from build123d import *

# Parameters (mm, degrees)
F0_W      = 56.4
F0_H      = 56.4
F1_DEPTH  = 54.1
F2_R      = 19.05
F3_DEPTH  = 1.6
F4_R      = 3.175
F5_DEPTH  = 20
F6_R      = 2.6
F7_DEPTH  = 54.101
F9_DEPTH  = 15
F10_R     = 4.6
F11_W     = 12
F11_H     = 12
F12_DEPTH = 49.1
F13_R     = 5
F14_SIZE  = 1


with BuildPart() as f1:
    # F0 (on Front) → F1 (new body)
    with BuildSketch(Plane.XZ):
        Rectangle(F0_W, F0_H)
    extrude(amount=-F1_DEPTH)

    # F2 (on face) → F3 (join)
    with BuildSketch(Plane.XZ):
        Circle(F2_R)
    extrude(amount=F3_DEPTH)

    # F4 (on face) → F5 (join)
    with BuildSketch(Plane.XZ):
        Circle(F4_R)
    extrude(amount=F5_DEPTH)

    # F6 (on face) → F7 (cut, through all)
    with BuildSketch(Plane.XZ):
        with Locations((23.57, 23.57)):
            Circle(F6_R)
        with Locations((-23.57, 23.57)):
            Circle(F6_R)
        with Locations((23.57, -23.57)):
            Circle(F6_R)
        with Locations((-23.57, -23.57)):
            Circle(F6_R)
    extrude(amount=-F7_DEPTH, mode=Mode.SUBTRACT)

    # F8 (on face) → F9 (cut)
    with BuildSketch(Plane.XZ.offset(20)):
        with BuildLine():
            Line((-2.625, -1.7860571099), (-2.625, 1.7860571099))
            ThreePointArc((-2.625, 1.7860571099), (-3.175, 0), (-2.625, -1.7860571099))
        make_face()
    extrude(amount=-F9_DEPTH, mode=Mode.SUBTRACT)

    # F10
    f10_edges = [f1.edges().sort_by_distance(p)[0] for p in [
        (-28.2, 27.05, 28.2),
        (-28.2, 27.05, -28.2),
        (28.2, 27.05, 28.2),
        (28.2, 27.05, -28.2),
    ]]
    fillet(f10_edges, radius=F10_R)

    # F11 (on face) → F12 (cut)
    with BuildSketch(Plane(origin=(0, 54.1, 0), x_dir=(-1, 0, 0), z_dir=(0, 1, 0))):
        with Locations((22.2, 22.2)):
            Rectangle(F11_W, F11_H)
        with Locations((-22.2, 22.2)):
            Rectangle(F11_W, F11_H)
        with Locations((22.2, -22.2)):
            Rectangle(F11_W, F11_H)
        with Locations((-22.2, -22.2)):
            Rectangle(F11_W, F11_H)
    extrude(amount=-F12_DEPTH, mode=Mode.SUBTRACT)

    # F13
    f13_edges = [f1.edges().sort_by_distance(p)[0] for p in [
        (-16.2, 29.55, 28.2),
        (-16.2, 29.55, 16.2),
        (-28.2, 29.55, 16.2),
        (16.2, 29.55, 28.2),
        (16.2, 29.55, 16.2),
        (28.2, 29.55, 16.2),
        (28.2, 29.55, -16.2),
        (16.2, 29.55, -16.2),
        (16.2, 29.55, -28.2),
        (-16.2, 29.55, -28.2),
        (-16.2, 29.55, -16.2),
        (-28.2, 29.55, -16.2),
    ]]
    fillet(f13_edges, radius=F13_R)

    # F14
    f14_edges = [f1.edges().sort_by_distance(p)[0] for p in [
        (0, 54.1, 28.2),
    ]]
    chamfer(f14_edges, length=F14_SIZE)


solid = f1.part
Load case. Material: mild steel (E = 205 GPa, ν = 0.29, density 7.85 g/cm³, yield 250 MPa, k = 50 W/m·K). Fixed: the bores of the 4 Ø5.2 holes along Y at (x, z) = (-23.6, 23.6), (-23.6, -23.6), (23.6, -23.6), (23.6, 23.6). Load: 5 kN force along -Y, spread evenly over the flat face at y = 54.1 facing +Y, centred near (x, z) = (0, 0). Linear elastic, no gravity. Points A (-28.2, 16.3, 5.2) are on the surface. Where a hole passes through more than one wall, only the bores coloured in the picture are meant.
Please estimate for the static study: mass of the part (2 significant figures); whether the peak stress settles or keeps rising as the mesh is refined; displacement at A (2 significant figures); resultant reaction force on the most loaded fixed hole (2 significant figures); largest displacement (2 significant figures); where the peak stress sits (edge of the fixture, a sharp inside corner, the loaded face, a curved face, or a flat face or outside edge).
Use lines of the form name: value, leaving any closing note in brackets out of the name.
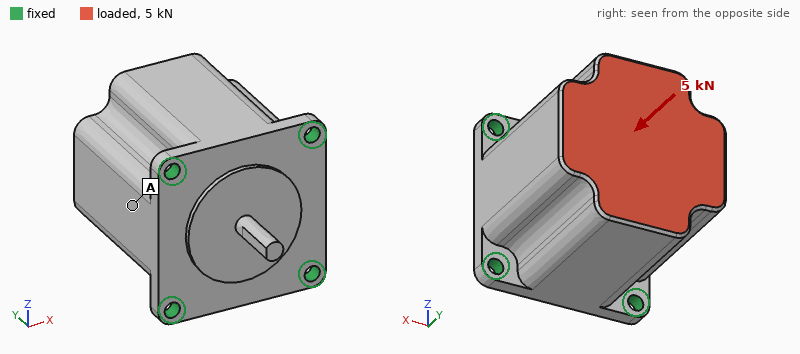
mass of the part: 1.1 kg
whether the peak stress settles or keeps rising as the mesh is refined: keeps rising
displacement at A: 3.2 µm
resultant reaction force on the most loaded fixed hole: 1.3 kN
largest displacement: 3.6 µm
where the peak stress sits: edge of the fixture
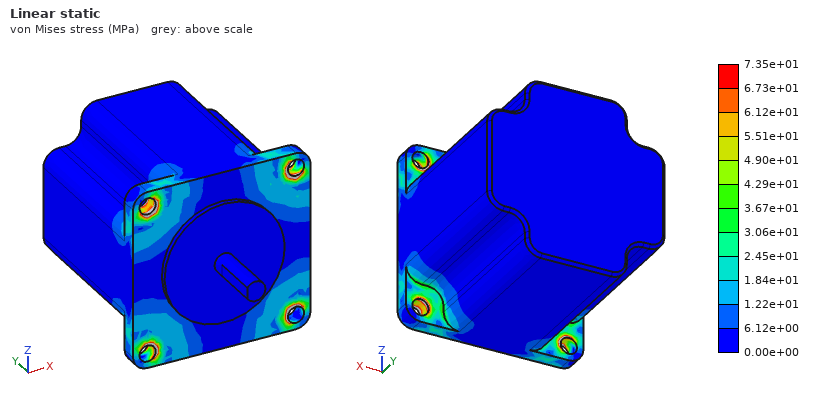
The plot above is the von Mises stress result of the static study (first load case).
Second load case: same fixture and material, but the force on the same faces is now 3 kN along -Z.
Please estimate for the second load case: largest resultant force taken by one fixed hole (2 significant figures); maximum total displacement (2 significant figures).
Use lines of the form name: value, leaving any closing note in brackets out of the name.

largest resultant force taken by one fixed hole: 2.0 kN
maximum total displacement: 15 µm
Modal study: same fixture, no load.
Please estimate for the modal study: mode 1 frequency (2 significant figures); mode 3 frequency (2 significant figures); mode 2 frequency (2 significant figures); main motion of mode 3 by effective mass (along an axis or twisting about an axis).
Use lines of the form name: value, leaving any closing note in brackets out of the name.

mode 1 frequency: 3700 Hz
mode 3 frequency: 5900 Hz
mode 2 frequency: 3700 Hz
main motion of mode 3 by effective mass: along Y
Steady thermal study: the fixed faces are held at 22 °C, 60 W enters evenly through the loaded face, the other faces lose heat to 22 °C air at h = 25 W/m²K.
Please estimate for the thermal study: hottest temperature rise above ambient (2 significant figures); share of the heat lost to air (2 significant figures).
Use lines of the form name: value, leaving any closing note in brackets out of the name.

hottest temperature rise above ambient: 47 K
share of the heat lost to air: 19 %
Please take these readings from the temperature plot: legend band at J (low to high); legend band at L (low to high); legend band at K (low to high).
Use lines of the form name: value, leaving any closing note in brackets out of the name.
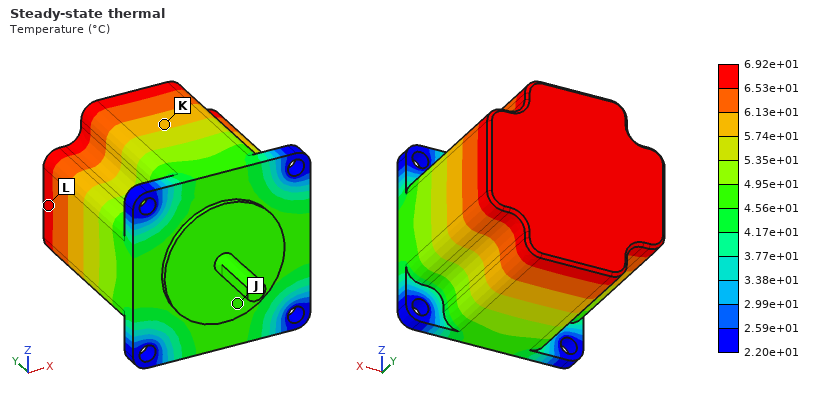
legend band at J: 4.56e+01 to 4.95e+01 °C
legend band at L: 6.53e+01 to 6.92e+01 °C
legend band at K: 5.74e+01 to 6.13e+01 °C
